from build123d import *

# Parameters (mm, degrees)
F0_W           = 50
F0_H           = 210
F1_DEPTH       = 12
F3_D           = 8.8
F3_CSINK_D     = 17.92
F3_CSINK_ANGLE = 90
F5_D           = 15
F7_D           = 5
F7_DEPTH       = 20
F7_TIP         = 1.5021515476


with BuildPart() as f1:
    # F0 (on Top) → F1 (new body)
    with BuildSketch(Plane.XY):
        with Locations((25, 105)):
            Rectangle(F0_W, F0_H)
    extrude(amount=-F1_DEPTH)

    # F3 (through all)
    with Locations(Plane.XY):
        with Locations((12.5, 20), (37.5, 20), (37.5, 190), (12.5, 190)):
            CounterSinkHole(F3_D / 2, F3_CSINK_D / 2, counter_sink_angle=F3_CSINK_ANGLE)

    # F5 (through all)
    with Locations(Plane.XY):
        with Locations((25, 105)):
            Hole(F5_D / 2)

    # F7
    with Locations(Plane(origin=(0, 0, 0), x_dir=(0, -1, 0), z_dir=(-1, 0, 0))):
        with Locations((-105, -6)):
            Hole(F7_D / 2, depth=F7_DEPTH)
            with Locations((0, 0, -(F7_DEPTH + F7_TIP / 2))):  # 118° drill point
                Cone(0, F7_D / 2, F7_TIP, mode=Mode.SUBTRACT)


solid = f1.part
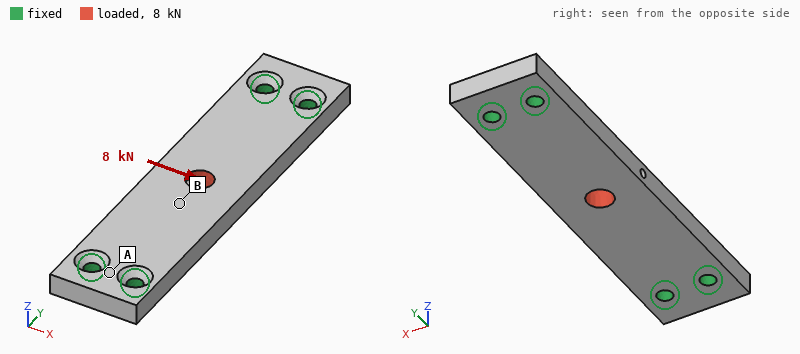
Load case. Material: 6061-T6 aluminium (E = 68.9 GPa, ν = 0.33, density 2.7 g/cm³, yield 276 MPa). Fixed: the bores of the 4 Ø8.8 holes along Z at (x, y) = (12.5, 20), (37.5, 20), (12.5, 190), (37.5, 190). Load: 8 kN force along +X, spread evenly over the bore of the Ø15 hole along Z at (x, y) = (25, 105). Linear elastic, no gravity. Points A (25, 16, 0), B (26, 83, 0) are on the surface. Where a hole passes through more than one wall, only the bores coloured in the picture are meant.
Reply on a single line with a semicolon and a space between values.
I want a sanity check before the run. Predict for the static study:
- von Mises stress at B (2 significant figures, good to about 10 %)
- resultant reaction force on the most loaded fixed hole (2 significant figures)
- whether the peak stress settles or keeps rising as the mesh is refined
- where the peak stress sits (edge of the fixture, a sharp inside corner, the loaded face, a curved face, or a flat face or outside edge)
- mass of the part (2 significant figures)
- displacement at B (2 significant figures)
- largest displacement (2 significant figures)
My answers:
16 MPa; 5.6 kN; keeps rising; edge of the fixture; 320 g; 43 µm; 56 µm
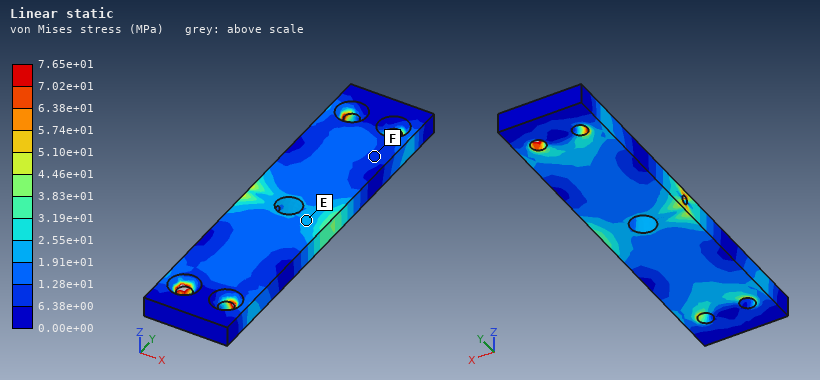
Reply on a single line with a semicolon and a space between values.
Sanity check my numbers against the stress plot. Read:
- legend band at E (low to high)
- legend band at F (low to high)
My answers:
1.91e+01 to 2.55e+01 MPa; 6.38e+00 to 1.28e+01 MPa
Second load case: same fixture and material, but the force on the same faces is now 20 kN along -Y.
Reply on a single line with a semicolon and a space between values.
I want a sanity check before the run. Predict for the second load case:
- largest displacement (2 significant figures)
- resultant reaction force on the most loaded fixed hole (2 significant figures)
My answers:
26 µm; 5.1 kN
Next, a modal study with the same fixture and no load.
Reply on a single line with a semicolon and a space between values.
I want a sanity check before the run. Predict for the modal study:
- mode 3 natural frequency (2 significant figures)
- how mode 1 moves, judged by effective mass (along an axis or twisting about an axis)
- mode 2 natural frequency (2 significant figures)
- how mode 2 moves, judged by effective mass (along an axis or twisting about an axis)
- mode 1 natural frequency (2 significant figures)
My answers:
5200 Hz; along Z; 4400 Hz; twisting about Y; 2000 Hz
